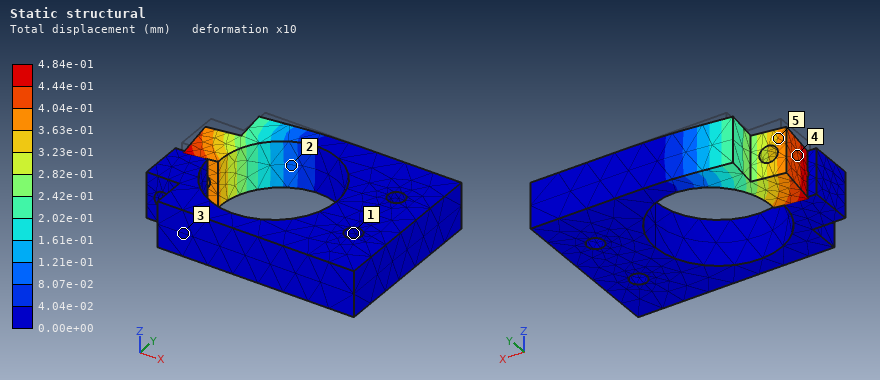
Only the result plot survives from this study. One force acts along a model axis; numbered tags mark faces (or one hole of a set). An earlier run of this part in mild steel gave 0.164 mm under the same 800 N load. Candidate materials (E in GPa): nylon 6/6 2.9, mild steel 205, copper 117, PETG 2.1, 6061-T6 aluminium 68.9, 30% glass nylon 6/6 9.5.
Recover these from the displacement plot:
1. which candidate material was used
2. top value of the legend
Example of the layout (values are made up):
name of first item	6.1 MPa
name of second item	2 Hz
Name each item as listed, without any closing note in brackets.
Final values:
which candidate material was used	6061-T6 aluminium
top value of the legend	4.84e-01 mm
